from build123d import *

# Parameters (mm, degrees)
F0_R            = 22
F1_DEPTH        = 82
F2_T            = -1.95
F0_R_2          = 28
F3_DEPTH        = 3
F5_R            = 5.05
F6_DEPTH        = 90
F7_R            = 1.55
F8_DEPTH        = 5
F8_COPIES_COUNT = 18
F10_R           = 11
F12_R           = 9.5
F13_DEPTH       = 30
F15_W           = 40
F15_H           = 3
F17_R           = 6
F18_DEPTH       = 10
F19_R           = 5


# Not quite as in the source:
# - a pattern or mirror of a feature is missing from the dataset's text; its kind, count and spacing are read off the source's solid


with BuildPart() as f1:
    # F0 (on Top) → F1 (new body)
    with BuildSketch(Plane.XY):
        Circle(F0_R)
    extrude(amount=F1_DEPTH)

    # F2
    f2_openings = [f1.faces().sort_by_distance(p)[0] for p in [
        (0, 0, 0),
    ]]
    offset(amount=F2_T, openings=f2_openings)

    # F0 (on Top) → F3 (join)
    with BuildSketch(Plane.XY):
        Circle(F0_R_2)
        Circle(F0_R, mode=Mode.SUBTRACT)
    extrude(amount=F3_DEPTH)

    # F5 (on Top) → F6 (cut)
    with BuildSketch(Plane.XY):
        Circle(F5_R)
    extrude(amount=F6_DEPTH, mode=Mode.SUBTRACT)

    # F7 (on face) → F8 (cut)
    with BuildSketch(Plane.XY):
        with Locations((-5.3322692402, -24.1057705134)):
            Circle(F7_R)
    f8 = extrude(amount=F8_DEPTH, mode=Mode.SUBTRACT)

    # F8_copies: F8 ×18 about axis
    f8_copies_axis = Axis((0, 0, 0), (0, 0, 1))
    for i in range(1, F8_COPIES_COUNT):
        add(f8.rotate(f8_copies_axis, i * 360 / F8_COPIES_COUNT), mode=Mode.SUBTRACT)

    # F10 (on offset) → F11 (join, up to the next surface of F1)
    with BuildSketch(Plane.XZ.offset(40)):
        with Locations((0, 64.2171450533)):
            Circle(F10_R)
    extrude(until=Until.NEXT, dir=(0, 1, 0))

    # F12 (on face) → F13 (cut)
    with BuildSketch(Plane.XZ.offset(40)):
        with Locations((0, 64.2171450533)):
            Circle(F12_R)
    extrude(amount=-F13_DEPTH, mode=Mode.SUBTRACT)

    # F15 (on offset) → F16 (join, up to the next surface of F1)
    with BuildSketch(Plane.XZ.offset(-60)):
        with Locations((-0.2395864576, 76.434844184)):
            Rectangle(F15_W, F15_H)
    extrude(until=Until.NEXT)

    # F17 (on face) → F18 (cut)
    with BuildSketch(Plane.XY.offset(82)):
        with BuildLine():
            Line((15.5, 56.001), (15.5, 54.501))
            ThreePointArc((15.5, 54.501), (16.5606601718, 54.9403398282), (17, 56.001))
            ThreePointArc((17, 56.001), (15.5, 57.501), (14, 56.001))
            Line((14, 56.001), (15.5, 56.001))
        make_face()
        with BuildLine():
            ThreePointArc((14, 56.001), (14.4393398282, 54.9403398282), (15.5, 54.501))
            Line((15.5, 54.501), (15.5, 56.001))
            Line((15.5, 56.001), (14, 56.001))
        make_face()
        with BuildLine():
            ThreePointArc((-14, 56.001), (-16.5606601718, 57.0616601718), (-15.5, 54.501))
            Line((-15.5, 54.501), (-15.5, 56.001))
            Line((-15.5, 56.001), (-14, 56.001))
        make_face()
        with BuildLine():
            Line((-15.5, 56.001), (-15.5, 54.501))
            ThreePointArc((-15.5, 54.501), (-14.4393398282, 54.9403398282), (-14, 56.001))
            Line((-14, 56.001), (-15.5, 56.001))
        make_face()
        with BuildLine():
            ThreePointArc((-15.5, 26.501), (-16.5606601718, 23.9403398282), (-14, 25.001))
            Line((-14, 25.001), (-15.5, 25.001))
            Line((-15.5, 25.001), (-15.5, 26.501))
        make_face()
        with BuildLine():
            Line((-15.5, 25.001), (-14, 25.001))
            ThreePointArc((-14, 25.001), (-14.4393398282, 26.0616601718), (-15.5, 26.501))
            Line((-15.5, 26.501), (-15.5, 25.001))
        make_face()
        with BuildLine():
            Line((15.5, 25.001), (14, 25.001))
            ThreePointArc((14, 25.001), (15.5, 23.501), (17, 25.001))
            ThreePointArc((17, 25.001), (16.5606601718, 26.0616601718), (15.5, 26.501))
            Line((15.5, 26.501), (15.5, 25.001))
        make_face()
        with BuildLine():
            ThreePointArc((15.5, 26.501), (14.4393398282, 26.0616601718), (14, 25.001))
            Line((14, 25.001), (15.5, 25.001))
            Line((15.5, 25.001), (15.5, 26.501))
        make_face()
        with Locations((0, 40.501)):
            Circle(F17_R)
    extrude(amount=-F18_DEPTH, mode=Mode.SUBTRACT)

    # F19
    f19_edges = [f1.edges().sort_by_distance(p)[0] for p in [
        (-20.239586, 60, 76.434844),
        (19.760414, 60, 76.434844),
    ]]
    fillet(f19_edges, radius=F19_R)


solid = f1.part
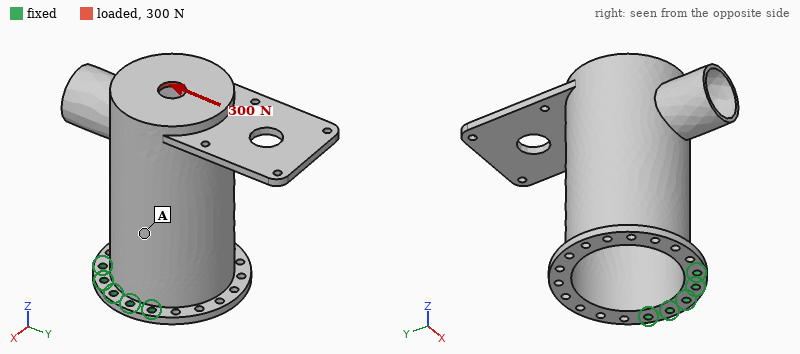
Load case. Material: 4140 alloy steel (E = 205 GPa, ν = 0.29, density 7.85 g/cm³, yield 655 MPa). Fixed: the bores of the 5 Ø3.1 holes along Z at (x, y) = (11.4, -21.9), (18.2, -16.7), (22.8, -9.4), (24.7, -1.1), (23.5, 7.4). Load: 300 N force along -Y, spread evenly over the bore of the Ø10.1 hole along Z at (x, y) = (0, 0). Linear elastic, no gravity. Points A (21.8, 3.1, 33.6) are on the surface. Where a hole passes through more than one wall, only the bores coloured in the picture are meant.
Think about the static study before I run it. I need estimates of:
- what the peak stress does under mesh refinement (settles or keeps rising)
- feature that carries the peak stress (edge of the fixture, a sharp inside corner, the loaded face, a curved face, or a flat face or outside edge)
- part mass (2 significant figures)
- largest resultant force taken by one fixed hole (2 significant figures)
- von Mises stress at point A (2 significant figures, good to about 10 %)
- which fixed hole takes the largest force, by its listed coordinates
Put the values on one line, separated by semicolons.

keeps rising; edge of the fixture; 250 g; 1.2 kN; 9.9 MPa; (23.5, 7.4)
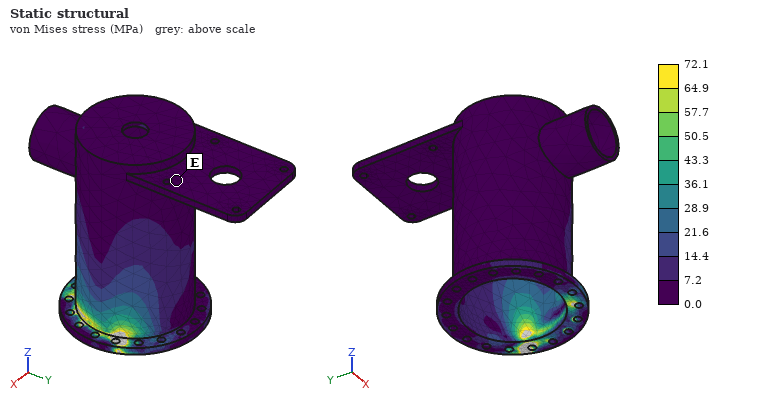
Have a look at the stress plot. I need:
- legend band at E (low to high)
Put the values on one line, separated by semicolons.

0.0 to 7.2 MPa
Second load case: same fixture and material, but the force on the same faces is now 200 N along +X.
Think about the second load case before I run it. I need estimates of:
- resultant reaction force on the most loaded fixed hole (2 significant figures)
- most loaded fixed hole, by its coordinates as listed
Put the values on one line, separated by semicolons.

1.1 kN; (11.4, -21.9)
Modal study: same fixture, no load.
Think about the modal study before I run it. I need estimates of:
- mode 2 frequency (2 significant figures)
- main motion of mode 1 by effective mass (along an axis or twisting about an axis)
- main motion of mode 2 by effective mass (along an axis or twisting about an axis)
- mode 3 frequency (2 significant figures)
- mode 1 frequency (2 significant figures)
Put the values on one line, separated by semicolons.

1100 Hz; along X; along Y; 1400 Hz; 420 Hz
